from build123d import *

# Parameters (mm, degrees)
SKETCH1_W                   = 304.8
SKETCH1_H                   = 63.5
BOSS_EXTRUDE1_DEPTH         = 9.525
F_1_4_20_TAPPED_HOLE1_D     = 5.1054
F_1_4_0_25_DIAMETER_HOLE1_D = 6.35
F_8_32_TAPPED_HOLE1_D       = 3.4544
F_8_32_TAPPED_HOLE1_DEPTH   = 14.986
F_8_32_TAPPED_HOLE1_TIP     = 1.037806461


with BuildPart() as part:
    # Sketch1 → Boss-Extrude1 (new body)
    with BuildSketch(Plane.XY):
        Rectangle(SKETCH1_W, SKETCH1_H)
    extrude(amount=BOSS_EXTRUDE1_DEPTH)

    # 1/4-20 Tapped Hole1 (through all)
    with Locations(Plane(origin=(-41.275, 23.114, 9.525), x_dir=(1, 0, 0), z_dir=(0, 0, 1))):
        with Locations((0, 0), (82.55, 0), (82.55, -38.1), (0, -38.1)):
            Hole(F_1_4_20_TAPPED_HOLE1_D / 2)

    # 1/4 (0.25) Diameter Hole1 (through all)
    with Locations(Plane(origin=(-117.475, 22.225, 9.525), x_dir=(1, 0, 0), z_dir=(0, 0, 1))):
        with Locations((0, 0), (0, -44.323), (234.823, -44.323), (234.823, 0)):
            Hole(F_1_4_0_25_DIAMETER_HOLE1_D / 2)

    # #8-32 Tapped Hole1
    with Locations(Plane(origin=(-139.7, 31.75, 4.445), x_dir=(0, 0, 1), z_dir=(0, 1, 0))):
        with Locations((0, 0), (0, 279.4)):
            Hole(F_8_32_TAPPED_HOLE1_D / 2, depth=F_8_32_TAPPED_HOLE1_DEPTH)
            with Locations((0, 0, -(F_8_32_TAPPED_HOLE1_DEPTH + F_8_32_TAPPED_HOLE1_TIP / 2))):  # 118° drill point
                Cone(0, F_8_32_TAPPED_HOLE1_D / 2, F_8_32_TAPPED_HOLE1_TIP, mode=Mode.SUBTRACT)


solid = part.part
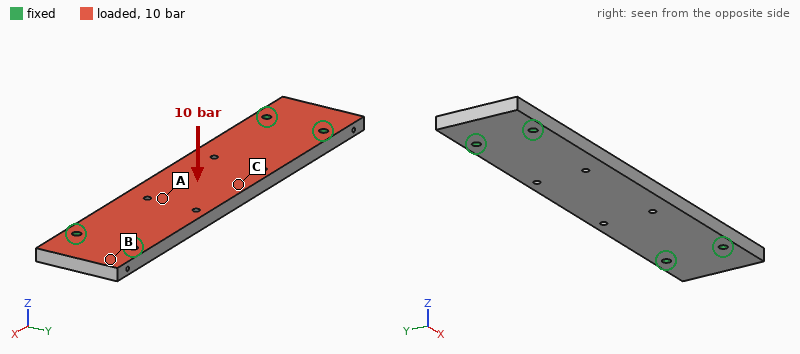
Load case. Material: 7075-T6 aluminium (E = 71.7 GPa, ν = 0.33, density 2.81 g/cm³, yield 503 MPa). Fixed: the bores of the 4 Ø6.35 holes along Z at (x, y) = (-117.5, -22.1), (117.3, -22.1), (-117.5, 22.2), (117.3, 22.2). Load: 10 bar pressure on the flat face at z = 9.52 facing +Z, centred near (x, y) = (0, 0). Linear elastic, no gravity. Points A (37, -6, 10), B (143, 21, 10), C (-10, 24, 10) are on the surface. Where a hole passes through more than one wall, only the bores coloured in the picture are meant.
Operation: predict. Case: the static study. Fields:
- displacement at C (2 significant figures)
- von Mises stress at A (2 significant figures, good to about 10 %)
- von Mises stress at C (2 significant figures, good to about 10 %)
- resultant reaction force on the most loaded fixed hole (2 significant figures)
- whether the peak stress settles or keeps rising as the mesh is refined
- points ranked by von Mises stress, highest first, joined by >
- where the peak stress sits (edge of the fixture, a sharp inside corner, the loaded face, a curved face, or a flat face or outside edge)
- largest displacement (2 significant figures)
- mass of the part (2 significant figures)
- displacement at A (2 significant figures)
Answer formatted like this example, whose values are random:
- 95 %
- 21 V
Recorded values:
- 1.6 mm
- 110 MPa
- 150 MPa
- 4.8 kN
- keeps rising
- C > A > B
- edge of the fixture
- 1.6 mm
- 510 g
- 1.3 mm
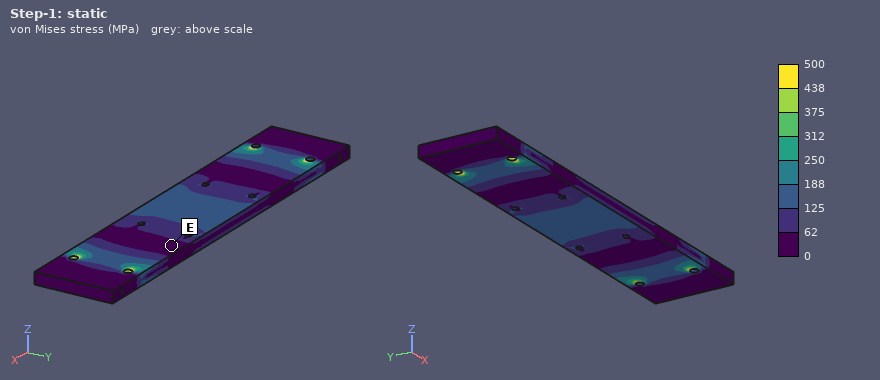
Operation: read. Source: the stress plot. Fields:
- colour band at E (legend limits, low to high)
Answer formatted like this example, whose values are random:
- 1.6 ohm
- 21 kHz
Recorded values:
- 0 to 62 MPa
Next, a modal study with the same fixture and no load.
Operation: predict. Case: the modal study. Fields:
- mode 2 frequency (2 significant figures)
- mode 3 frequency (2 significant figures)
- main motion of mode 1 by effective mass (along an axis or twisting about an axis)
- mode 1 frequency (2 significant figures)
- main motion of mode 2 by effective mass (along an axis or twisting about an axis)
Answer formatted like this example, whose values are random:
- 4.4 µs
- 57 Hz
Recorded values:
- 2200 Hz
- 2400 Hz
- along Z
- 870 Hz
- twisting about X
